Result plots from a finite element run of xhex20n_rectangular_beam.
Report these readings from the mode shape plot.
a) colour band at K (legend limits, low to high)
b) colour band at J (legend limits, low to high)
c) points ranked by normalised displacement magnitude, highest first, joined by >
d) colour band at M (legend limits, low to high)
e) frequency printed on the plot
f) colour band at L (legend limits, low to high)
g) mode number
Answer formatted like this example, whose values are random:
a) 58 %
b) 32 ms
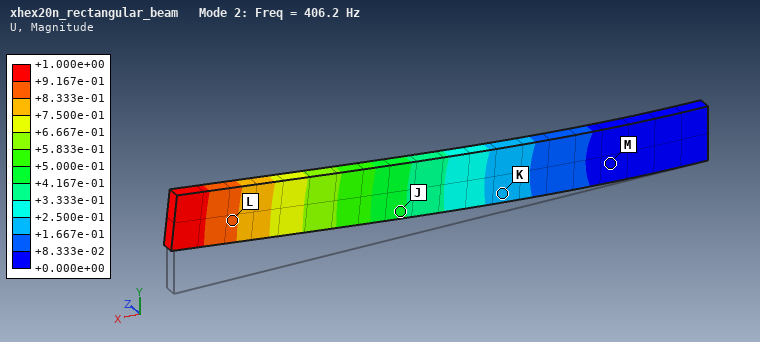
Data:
a) +1.667e-01 to +2.500e-01
b) +4.167e-01 to +5.000e-01
c) L > J > K > M
d) +0.000e+00 to +8.333e-02
e) 406.2 Hz
f) +8.333e-01 to +9.167e-01
g) 2
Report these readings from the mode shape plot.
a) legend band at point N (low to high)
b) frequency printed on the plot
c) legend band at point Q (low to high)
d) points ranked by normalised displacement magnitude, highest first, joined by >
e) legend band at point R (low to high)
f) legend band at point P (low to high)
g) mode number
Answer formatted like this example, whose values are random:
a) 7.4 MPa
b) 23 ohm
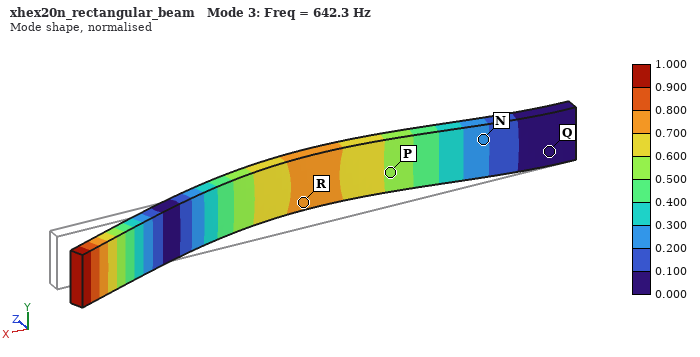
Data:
a) 0.200 to 0.300
b) 642.3 Hz
c) 0.000 to 0.100
d) R > P > N > Q
e) 0.700 to 0.800
f) 0.500 to 0.600
g) 3
